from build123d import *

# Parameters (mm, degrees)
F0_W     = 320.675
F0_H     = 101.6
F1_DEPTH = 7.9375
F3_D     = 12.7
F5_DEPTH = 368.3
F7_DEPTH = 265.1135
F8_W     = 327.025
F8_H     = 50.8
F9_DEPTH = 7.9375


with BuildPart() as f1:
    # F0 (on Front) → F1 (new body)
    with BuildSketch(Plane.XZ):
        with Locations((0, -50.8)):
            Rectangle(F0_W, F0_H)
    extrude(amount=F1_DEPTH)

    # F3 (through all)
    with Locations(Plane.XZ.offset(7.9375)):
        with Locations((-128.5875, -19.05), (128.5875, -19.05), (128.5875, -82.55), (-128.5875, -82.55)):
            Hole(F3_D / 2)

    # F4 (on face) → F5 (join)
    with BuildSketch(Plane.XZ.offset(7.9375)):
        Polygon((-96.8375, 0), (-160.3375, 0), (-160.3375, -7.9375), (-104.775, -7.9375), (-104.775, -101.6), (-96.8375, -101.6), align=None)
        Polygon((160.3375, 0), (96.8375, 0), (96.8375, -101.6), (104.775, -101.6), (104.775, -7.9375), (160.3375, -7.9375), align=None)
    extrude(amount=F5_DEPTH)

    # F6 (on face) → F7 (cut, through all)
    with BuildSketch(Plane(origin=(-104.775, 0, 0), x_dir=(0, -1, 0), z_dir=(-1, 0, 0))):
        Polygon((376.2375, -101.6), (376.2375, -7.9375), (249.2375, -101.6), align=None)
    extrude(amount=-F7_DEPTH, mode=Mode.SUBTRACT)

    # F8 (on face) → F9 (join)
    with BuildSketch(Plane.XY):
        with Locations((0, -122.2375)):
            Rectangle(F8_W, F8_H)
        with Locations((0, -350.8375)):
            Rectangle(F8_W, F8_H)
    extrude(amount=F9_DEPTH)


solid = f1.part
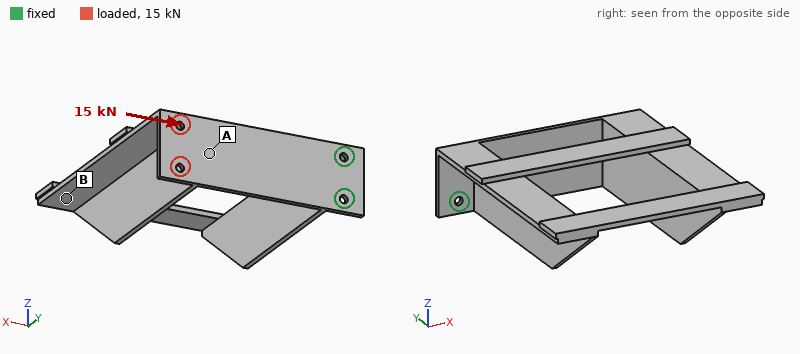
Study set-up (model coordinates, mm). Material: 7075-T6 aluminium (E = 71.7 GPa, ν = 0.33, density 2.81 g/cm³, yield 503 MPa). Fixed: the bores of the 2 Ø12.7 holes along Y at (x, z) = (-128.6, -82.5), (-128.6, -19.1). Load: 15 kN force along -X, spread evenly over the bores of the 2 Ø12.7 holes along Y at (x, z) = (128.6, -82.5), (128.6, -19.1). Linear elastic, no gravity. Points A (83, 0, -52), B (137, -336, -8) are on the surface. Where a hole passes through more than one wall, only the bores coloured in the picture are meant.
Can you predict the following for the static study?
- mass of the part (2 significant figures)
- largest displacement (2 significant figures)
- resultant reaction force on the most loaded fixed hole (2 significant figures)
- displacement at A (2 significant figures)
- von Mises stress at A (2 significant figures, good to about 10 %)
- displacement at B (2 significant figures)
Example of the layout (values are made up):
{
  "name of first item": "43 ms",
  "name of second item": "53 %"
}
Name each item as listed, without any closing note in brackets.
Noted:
{
  "mass of the part": "3.8 kg",
  "largest displacement": "0.10 mm",
  "resultant reaction force on the most loaded fixed hole": "7.6 kN",
  "displacement at A": "0.071 mm",
  "von Mises stress at A": "17 MPa",
  "displacement at B": "0.074 mm"
}
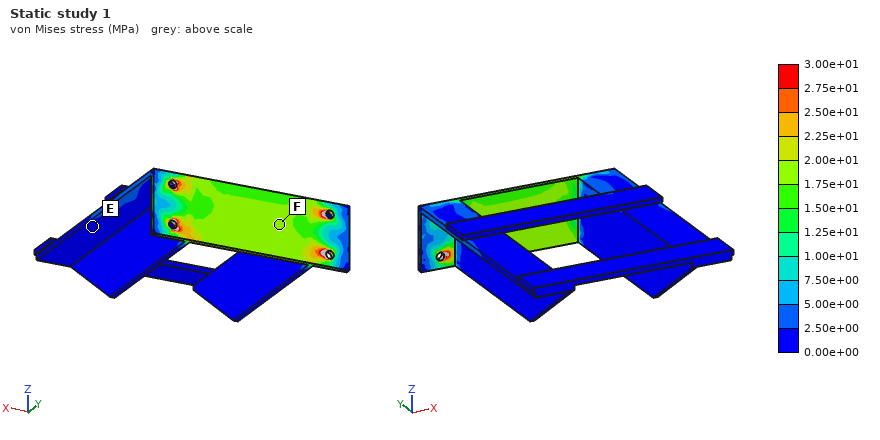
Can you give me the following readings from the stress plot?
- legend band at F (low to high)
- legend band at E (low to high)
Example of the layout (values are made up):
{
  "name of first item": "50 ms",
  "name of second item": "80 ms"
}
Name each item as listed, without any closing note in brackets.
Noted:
{
  "legend band at F": "1.75e+01 to 2.00e+01 MPa",
  "legend band at E": "0.00e+00 to 2.50e+00 MPa"
}
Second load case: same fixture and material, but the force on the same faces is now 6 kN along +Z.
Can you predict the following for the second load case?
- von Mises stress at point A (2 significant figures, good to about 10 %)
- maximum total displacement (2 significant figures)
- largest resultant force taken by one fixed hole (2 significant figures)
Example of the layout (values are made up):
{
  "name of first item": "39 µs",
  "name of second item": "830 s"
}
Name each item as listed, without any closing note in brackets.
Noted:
{
  "von Mises stress at point A": "19 MPa",
  "maximum total displacement": "0.92 mm",
  "largest resultant force taken by one fixed hole": "22 kN"
}
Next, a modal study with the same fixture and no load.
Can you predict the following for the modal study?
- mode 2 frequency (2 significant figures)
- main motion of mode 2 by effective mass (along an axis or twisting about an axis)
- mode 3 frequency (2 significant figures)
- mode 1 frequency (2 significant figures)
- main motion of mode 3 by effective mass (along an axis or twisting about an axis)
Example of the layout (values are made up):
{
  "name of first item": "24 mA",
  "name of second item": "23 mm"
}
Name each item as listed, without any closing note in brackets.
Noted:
{
  "mode 2 frequency": "72 Hz",
  "main motion of mode 2 by effective mass": "along Z",
  "mode 3 frequency": "240 Hz",
  "mode 1 frequency": "58 Hz",
  "main motion of mode 3 by effective mass": "along Z"
}
